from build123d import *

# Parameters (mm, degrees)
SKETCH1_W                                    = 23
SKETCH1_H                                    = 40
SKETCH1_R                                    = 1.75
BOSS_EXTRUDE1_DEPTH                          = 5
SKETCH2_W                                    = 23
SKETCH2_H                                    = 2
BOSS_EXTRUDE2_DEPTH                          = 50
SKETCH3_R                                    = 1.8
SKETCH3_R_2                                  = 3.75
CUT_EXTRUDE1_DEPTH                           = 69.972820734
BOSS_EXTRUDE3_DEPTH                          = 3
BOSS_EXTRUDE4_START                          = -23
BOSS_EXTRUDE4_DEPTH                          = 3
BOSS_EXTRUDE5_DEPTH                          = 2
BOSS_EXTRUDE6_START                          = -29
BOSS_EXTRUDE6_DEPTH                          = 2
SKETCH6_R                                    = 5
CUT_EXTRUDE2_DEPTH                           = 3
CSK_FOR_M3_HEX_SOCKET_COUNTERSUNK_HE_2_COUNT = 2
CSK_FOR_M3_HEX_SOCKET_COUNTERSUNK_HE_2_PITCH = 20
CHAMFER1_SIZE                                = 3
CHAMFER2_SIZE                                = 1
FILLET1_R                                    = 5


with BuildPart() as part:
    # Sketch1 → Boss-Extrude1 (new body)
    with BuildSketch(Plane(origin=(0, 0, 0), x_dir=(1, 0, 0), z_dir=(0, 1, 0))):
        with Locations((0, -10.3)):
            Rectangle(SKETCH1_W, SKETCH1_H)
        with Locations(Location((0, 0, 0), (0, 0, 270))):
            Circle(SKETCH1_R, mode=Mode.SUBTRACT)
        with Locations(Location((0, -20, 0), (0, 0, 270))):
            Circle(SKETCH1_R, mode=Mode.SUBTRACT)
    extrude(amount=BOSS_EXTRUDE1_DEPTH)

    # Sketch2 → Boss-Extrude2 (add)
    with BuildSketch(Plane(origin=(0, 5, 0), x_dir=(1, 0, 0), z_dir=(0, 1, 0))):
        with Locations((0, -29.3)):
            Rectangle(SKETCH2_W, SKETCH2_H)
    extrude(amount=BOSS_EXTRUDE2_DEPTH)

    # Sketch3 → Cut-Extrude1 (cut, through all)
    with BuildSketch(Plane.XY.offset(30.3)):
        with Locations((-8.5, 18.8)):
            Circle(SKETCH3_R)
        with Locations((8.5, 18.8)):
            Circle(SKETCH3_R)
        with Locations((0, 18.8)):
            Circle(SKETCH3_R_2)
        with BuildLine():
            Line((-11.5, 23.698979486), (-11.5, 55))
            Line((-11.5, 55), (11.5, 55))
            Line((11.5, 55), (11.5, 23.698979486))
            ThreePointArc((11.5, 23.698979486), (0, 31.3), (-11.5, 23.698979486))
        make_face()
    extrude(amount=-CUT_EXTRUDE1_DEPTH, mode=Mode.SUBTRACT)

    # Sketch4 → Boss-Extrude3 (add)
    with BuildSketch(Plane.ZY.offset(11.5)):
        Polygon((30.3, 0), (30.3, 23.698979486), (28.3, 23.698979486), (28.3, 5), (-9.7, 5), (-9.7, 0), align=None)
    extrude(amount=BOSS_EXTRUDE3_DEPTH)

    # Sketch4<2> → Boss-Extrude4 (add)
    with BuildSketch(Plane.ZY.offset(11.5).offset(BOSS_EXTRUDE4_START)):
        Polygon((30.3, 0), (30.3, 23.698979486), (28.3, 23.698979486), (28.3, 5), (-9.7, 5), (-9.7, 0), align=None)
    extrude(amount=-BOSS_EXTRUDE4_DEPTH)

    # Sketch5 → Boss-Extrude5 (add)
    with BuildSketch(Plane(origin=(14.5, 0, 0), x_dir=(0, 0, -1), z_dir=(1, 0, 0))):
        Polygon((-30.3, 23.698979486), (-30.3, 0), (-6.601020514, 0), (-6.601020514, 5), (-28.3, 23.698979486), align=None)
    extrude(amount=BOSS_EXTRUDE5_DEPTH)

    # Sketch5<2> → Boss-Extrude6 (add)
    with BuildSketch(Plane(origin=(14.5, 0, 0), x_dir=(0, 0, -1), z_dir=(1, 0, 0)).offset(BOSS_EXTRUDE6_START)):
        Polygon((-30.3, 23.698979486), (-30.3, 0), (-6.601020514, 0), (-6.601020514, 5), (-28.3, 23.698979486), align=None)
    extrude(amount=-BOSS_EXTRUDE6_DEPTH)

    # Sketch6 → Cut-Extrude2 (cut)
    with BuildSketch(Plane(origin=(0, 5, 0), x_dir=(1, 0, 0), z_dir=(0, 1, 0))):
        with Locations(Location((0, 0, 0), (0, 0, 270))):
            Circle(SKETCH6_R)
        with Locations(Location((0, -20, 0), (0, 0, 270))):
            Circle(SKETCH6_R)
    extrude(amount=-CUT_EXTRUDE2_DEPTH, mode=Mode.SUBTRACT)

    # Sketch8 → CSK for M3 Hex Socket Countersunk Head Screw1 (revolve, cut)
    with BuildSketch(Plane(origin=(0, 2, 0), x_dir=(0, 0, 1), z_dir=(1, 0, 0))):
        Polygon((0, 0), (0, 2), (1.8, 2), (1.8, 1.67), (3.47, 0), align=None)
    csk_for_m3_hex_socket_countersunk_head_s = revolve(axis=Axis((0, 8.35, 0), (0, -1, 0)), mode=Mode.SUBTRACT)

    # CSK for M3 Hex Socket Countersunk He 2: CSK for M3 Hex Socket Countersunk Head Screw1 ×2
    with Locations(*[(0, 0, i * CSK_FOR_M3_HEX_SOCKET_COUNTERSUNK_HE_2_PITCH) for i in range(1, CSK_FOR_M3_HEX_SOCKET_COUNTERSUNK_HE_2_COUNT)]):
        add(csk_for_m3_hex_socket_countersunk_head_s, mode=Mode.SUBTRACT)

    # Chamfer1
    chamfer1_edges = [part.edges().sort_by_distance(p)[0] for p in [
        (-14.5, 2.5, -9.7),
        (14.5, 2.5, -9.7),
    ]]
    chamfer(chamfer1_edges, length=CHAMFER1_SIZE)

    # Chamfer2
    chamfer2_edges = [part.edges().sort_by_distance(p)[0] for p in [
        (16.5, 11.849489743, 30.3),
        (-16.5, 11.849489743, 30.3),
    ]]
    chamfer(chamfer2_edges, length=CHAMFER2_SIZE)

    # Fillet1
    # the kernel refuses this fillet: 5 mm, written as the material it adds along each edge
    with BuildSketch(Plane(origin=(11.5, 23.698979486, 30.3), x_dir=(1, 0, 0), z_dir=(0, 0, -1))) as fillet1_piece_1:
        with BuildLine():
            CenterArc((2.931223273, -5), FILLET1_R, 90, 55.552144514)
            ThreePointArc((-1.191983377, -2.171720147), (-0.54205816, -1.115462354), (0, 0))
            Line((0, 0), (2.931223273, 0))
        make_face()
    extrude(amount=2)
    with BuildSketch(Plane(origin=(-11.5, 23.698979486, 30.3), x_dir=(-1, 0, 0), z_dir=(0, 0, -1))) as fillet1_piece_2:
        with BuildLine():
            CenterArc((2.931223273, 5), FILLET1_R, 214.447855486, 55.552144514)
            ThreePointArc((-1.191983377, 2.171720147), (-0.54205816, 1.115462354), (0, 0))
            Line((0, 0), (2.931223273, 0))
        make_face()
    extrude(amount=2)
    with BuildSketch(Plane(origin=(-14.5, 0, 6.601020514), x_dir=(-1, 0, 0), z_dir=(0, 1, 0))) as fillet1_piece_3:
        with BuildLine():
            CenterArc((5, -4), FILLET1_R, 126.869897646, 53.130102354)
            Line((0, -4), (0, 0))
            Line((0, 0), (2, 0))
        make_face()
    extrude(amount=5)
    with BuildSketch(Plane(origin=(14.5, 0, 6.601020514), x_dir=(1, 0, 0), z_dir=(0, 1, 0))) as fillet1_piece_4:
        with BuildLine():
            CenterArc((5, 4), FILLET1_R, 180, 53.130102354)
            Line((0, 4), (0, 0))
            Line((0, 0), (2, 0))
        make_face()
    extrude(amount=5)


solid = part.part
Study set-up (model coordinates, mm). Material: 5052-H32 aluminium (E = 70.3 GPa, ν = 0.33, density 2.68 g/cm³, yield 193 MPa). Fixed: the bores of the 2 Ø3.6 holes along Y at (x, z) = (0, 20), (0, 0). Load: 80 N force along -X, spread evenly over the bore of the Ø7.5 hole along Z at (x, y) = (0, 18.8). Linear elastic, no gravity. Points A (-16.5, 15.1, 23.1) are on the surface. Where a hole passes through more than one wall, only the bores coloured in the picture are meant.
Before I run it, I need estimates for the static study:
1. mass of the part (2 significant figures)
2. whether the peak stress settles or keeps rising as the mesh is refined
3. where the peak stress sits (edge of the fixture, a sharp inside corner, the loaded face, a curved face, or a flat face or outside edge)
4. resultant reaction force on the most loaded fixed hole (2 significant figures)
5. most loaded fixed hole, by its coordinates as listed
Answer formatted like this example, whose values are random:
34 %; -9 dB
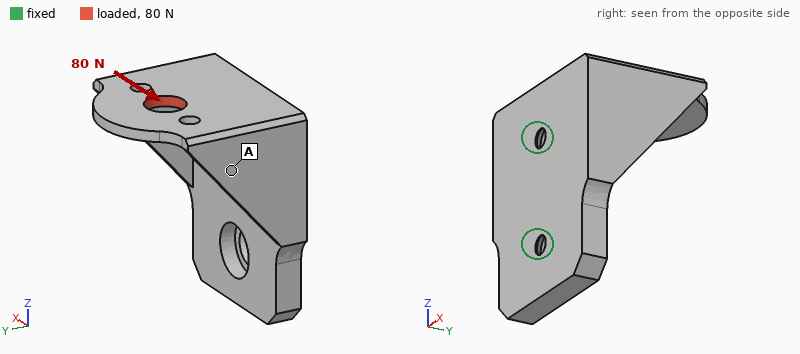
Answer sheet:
21 g; keeps rising; edge of the fixture; 110 N; (0, 20)
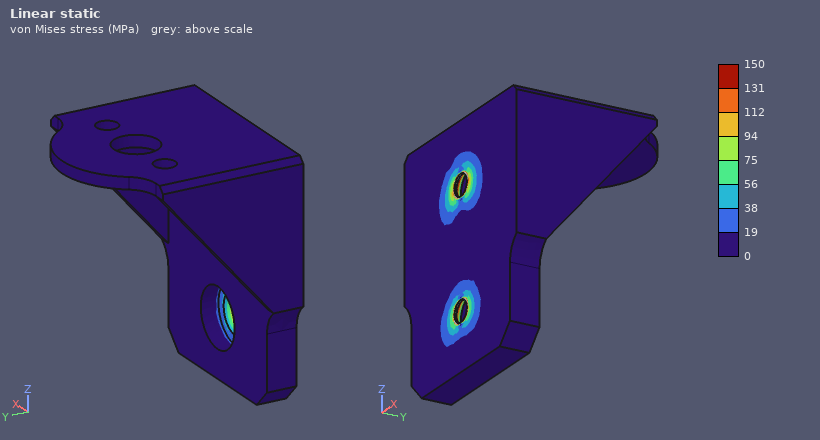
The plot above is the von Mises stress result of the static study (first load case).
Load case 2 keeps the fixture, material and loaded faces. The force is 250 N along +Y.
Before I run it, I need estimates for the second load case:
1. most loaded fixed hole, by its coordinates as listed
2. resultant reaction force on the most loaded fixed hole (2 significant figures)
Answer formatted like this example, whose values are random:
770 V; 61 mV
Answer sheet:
(0, 20); 370 N
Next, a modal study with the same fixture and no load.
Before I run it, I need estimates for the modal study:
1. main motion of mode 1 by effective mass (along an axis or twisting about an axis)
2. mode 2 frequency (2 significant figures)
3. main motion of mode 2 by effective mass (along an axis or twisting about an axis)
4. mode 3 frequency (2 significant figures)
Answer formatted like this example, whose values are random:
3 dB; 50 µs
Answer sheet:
along X; 4800 Hz; along Z; 7200 Hz
